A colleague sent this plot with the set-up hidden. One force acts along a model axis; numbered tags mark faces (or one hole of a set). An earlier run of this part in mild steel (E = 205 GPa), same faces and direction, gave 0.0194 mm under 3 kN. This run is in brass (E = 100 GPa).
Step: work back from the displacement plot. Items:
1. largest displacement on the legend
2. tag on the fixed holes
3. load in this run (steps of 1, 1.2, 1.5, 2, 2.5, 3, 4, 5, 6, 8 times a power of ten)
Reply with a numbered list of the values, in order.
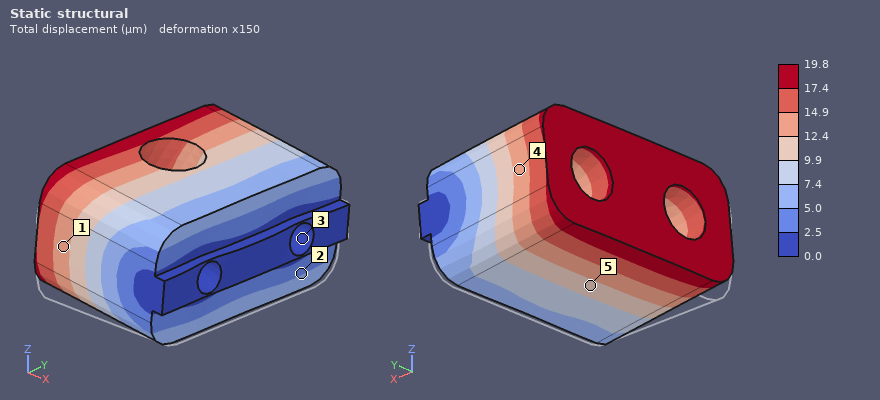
1. 19.8 µm
2. 3
3. 1.5 kN
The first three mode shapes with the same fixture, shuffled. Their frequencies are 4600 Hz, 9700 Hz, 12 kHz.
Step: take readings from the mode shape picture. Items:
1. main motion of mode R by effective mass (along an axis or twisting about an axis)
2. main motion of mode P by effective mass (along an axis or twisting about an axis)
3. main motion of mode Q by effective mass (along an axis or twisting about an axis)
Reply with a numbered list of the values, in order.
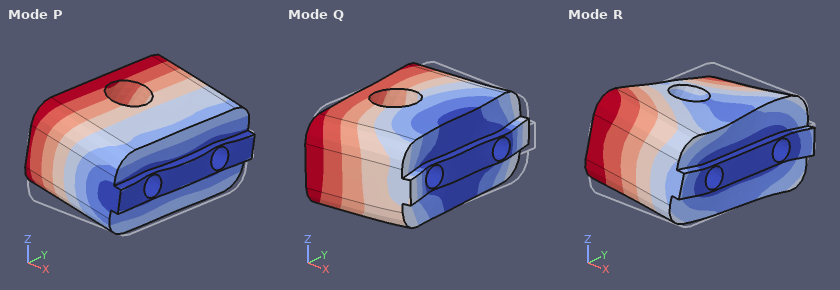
1. twisting about X
2. along Z
3. along Y
